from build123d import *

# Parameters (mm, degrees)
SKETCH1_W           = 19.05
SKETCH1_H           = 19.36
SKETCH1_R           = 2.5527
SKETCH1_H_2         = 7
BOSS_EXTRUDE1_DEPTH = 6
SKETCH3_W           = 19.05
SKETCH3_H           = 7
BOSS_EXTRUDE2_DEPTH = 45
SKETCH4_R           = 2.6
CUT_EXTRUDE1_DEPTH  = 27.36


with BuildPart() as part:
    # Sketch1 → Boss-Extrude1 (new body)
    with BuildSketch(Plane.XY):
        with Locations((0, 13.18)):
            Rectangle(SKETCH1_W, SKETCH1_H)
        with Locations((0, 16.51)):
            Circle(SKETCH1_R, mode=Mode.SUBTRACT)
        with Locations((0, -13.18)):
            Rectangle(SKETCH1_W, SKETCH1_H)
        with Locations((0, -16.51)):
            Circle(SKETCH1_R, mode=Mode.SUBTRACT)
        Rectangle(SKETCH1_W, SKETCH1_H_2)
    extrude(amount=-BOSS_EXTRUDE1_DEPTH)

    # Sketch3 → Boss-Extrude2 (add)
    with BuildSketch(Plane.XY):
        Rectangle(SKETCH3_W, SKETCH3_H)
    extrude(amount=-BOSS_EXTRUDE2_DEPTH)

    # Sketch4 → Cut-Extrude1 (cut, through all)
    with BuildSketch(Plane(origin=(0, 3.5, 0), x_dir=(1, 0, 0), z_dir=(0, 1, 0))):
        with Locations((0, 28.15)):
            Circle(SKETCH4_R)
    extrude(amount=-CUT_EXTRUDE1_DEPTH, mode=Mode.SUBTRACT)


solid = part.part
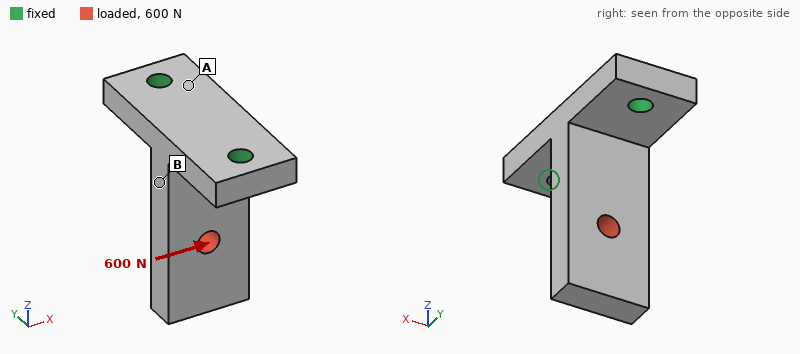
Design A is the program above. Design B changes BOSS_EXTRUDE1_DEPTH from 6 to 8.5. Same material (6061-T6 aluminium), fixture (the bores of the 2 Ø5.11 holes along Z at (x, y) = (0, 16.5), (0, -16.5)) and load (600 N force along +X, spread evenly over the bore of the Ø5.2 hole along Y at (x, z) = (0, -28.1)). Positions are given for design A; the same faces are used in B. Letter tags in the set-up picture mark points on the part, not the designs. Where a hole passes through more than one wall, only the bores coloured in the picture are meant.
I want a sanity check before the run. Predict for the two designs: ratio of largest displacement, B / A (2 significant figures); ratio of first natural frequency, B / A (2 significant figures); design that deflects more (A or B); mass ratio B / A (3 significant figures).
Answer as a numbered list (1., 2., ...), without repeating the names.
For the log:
1. 0.49
2. 1.2
3. A
4. 1.17
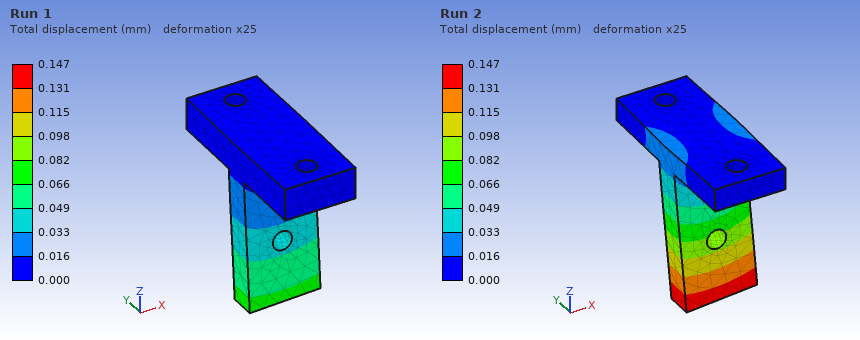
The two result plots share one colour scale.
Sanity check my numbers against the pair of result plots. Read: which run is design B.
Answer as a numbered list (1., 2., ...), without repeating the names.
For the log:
1. Run 1
